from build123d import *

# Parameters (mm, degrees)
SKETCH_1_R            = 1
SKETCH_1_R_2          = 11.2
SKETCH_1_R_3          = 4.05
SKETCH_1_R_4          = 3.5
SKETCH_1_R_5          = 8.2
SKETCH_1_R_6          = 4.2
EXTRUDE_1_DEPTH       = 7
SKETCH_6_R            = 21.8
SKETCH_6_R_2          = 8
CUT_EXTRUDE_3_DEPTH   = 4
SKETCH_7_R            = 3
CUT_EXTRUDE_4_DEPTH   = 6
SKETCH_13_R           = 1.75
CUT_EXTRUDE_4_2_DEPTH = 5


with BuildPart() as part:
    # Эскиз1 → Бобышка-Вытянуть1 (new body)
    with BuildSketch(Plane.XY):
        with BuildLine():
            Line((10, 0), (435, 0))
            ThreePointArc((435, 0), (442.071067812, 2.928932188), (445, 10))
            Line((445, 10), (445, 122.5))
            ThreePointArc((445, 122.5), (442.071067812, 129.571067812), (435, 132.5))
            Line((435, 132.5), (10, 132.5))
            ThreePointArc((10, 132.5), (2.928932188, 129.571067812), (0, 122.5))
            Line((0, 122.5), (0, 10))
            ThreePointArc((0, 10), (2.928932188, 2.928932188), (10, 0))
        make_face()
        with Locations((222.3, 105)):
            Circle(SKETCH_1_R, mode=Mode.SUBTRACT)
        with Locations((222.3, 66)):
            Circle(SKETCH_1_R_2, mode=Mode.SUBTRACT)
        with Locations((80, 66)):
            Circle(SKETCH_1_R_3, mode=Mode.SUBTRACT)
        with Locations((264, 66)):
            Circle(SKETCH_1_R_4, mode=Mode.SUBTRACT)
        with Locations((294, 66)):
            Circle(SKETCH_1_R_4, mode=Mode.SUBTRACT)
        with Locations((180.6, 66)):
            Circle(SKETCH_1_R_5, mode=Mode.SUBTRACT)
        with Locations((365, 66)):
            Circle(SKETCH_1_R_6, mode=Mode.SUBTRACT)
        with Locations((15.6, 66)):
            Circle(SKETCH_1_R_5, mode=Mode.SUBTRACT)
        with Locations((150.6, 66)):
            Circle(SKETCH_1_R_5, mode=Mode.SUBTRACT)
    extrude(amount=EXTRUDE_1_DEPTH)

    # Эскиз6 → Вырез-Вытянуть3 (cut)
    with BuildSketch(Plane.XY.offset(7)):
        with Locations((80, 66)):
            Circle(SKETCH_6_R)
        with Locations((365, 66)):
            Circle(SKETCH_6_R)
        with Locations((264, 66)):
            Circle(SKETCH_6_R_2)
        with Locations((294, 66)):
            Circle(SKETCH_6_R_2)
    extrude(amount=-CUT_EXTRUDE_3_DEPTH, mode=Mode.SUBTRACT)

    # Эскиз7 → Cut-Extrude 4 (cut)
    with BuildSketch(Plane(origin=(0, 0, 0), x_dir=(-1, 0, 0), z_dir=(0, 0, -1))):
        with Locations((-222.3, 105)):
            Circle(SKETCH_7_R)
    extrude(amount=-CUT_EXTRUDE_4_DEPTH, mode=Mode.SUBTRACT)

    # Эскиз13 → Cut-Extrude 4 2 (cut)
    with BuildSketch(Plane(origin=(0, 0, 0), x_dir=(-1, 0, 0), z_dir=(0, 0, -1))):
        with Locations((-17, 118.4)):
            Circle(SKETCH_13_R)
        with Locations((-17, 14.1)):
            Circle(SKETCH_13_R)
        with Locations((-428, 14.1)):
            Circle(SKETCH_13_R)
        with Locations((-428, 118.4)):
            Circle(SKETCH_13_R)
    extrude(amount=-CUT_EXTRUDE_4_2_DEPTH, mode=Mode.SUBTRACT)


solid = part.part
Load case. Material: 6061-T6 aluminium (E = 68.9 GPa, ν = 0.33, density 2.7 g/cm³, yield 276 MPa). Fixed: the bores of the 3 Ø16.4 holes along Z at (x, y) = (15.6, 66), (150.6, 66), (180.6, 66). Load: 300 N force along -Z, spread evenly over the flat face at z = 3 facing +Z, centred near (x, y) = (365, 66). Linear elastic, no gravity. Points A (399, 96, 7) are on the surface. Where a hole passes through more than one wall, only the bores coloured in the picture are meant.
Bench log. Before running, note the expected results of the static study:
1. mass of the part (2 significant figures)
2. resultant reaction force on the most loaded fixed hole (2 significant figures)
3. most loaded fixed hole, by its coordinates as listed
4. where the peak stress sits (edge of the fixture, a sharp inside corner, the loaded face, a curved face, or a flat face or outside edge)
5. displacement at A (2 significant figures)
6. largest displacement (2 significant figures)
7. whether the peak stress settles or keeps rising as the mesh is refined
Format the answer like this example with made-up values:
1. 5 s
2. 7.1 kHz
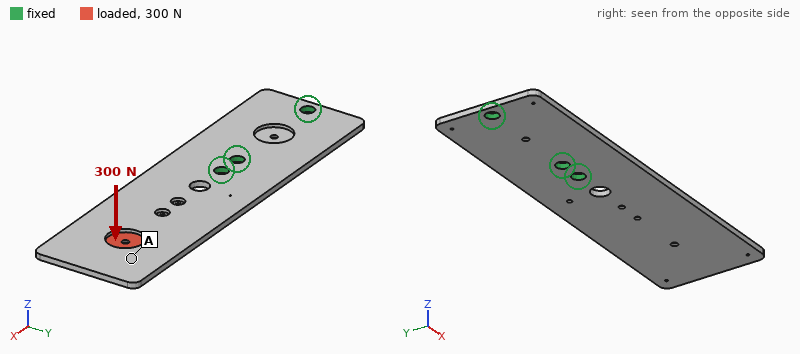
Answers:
1. 1.1 kg
2. 950 N
3. (180.6, 66)
4. edge of the fixture
5. 3.3 mm
6. 4.3 mm
7. keeps rising
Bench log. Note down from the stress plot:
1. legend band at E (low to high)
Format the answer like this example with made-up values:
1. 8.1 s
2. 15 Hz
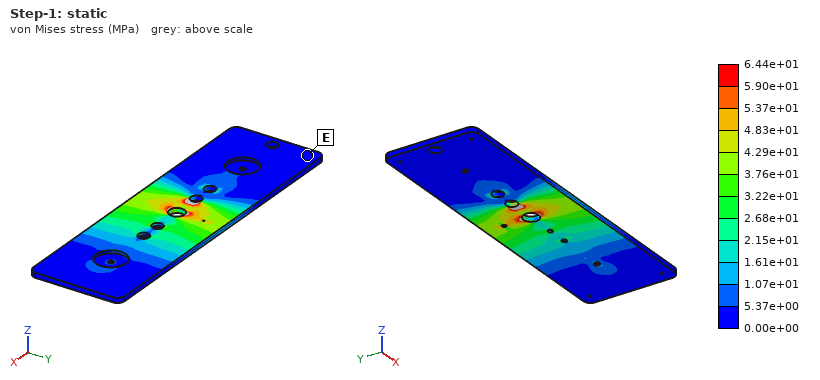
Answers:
1. 0.00e+00 to 5.37e+00 MPa
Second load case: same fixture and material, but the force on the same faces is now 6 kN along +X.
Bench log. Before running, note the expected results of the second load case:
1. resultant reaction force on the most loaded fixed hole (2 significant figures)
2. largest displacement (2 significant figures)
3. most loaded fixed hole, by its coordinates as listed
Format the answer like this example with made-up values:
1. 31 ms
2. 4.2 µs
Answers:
1. 3.4 kN
2. 0.34 mm
3. (180.6, 66)
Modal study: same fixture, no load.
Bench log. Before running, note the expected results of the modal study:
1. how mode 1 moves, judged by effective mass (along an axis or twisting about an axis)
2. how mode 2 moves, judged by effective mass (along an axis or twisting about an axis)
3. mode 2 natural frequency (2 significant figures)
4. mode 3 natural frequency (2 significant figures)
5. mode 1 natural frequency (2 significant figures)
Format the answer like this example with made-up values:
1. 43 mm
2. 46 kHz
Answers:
1. along Z
2. twisting about X
3. 300 Hz
4. 490 Hz
5. 80 Hz
